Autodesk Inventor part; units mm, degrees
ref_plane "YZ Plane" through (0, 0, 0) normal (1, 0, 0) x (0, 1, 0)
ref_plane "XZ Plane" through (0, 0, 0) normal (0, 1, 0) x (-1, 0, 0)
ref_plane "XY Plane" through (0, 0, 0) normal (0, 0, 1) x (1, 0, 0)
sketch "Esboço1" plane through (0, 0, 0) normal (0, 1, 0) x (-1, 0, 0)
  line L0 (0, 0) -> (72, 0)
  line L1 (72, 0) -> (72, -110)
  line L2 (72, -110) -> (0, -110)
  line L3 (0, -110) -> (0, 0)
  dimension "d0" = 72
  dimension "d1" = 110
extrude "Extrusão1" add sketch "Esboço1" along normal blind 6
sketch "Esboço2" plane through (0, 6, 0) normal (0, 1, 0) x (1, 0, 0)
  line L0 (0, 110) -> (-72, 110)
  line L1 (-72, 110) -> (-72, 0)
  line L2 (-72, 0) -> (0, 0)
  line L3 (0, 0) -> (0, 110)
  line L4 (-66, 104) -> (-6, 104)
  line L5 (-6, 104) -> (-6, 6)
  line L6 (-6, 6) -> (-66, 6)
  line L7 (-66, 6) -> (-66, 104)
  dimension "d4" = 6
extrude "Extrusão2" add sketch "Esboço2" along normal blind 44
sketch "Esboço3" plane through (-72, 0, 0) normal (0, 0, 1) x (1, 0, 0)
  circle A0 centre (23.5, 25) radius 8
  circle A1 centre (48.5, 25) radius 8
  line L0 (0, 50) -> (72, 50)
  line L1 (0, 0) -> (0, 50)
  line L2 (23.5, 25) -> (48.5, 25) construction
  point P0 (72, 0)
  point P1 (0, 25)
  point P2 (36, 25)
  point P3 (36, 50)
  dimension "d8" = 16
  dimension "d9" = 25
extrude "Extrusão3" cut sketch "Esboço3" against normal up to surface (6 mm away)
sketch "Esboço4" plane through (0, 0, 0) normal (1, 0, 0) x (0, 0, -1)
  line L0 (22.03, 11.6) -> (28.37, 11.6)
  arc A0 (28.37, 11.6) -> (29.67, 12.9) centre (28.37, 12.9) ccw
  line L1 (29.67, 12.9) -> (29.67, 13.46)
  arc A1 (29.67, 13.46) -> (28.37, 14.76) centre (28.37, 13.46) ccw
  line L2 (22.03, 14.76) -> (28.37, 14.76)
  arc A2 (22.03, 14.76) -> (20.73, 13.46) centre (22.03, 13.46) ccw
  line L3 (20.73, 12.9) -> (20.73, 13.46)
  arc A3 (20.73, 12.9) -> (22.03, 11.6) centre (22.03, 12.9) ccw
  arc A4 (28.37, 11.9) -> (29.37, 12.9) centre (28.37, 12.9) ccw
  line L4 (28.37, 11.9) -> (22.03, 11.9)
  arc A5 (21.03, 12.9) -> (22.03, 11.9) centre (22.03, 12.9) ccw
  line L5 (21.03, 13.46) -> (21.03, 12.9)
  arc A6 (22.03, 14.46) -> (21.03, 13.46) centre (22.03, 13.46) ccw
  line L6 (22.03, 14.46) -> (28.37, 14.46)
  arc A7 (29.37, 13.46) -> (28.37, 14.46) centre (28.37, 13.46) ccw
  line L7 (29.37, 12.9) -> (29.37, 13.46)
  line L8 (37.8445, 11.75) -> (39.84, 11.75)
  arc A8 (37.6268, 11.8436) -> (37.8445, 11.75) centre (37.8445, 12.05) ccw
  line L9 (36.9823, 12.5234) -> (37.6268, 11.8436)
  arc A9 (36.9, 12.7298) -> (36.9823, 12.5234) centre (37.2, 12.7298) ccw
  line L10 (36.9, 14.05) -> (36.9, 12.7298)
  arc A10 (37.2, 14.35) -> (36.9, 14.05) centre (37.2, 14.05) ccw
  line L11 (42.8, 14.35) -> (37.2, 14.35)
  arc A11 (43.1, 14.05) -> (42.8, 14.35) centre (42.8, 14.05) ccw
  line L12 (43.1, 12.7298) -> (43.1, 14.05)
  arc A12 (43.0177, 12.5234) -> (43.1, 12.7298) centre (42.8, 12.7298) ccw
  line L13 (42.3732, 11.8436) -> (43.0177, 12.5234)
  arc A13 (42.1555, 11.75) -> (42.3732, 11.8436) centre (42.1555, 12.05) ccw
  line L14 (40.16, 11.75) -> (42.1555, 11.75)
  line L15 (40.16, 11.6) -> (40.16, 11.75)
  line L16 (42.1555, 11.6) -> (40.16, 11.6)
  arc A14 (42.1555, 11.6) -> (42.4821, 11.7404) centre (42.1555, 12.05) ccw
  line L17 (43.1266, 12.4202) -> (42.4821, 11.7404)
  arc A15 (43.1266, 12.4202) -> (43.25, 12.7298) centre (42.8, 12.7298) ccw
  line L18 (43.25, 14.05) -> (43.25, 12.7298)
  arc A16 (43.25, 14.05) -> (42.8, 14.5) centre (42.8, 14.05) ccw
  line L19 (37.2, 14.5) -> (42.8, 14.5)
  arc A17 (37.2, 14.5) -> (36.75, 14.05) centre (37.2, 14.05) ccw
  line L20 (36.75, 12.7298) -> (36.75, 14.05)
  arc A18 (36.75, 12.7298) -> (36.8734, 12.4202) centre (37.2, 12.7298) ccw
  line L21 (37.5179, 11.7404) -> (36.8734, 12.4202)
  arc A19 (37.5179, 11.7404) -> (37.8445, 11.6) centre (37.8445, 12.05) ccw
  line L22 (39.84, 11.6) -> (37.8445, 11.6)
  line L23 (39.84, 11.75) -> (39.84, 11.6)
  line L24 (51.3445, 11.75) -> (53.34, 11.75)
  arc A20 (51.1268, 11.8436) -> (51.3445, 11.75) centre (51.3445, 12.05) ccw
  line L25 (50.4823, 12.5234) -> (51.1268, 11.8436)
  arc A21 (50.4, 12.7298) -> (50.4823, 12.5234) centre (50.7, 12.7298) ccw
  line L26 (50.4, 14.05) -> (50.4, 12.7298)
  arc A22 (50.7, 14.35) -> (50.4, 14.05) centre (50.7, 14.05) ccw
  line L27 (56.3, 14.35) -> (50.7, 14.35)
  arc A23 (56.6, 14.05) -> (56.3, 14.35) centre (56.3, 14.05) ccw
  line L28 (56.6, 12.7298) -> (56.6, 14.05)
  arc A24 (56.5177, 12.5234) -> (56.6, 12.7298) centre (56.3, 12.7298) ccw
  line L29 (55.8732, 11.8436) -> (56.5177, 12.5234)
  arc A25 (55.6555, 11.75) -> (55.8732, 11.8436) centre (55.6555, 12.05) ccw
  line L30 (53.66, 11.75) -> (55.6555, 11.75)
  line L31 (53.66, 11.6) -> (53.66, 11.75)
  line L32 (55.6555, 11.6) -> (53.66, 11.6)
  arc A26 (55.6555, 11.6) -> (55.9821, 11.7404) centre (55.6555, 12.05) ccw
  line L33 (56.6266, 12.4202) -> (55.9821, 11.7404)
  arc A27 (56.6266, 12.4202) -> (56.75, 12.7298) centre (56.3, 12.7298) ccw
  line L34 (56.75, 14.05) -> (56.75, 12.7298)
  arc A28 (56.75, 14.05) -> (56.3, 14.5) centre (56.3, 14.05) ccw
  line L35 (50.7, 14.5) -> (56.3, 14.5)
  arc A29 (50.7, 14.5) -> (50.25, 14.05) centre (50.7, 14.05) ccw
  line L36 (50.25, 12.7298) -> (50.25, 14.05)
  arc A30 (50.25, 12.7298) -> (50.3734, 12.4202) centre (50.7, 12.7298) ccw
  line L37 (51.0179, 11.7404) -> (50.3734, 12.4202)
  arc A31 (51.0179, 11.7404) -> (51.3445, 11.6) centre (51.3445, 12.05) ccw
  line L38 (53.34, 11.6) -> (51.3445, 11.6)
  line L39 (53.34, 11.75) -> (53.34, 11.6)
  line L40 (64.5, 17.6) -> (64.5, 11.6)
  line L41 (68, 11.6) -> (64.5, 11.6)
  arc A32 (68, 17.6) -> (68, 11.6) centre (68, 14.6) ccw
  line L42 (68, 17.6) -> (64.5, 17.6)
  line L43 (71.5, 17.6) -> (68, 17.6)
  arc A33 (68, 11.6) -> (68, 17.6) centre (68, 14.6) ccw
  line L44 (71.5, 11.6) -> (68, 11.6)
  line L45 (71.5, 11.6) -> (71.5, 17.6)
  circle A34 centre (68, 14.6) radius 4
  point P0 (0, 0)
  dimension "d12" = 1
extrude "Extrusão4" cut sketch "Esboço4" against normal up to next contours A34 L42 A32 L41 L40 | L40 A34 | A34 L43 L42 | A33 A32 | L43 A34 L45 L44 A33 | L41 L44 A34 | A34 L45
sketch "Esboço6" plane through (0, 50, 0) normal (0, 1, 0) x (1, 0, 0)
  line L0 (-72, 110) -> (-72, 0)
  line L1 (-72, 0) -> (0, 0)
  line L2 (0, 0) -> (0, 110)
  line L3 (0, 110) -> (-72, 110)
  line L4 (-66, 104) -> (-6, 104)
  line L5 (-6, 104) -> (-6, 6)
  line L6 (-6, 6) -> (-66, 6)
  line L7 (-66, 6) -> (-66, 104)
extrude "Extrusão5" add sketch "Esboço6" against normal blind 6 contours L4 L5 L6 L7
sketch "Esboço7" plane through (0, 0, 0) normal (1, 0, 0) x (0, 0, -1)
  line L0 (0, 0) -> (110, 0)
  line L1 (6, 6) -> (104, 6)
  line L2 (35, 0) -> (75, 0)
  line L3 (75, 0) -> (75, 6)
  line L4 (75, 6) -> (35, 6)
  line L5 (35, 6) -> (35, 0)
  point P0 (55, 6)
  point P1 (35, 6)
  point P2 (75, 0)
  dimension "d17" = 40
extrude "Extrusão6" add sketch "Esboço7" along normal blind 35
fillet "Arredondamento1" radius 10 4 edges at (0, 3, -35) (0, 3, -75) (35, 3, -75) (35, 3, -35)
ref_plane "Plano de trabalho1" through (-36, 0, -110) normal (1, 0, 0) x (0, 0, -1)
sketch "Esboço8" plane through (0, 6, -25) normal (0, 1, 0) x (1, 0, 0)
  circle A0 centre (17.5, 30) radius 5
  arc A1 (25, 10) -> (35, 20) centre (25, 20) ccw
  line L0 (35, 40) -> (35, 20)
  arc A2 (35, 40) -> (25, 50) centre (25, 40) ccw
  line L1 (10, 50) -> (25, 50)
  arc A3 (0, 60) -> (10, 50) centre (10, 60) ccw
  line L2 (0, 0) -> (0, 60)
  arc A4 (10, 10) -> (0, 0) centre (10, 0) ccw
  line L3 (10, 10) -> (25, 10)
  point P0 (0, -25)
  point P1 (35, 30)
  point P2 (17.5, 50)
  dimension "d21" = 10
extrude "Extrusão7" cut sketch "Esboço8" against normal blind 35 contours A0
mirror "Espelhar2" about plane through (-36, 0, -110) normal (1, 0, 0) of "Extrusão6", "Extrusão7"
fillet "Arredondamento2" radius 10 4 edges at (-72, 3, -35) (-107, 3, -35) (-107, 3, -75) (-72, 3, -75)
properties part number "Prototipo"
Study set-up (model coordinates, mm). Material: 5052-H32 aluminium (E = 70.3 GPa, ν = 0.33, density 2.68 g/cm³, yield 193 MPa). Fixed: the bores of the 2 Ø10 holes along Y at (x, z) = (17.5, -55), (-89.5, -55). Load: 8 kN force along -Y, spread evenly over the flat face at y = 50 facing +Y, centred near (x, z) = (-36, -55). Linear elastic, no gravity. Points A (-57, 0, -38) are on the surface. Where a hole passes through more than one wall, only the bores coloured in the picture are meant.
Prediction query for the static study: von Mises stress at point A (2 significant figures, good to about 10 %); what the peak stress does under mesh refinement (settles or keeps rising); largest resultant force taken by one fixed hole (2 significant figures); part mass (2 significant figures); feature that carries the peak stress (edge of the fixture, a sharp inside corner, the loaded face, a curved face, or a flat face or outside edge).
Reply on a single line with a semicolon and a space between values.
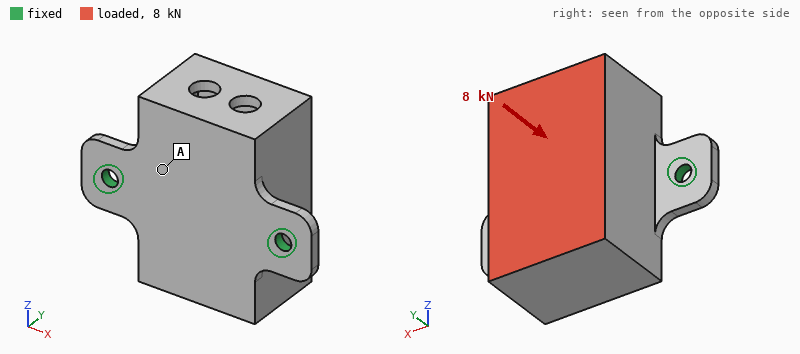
16 MPa; keeps rising; 4.1 kN; 500 g; edge of the fixture
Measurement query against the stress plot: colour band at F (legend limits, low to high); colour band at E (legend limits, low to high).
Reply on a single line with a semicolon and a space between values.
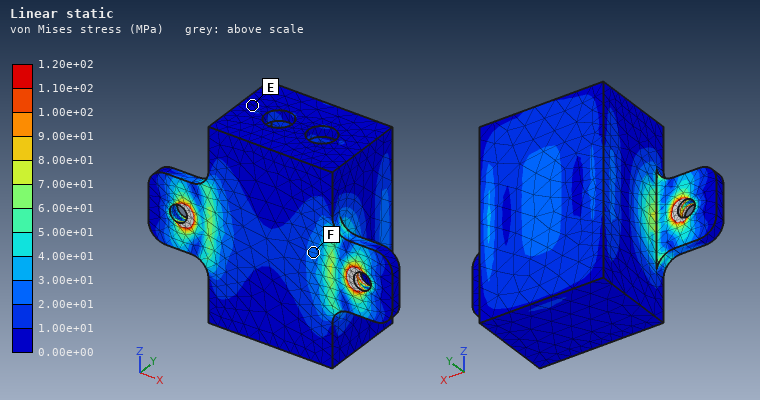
2.00e+01 to 3.00e+01 MPa; 0.00e+00 to 1.00e+01 MPa
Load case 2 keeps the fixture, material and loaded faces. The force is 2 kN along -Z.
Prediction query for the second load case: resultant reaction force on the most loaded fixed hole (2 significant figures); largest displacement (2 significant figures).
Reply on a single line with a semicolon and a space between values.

1.0 kN; 0.52 mm
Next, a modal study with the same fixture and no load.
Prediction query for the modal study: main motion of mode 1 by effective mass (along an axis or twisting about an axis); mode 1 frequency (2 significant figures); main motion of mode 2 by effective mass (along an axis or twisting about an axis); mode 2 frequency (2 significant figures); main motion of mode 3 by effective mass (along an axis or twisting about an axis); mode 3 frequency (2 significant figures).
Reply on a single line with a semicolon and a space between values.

along Z; 590 Hz; along Y; 2100 Hz; along X; 2300 Hz
